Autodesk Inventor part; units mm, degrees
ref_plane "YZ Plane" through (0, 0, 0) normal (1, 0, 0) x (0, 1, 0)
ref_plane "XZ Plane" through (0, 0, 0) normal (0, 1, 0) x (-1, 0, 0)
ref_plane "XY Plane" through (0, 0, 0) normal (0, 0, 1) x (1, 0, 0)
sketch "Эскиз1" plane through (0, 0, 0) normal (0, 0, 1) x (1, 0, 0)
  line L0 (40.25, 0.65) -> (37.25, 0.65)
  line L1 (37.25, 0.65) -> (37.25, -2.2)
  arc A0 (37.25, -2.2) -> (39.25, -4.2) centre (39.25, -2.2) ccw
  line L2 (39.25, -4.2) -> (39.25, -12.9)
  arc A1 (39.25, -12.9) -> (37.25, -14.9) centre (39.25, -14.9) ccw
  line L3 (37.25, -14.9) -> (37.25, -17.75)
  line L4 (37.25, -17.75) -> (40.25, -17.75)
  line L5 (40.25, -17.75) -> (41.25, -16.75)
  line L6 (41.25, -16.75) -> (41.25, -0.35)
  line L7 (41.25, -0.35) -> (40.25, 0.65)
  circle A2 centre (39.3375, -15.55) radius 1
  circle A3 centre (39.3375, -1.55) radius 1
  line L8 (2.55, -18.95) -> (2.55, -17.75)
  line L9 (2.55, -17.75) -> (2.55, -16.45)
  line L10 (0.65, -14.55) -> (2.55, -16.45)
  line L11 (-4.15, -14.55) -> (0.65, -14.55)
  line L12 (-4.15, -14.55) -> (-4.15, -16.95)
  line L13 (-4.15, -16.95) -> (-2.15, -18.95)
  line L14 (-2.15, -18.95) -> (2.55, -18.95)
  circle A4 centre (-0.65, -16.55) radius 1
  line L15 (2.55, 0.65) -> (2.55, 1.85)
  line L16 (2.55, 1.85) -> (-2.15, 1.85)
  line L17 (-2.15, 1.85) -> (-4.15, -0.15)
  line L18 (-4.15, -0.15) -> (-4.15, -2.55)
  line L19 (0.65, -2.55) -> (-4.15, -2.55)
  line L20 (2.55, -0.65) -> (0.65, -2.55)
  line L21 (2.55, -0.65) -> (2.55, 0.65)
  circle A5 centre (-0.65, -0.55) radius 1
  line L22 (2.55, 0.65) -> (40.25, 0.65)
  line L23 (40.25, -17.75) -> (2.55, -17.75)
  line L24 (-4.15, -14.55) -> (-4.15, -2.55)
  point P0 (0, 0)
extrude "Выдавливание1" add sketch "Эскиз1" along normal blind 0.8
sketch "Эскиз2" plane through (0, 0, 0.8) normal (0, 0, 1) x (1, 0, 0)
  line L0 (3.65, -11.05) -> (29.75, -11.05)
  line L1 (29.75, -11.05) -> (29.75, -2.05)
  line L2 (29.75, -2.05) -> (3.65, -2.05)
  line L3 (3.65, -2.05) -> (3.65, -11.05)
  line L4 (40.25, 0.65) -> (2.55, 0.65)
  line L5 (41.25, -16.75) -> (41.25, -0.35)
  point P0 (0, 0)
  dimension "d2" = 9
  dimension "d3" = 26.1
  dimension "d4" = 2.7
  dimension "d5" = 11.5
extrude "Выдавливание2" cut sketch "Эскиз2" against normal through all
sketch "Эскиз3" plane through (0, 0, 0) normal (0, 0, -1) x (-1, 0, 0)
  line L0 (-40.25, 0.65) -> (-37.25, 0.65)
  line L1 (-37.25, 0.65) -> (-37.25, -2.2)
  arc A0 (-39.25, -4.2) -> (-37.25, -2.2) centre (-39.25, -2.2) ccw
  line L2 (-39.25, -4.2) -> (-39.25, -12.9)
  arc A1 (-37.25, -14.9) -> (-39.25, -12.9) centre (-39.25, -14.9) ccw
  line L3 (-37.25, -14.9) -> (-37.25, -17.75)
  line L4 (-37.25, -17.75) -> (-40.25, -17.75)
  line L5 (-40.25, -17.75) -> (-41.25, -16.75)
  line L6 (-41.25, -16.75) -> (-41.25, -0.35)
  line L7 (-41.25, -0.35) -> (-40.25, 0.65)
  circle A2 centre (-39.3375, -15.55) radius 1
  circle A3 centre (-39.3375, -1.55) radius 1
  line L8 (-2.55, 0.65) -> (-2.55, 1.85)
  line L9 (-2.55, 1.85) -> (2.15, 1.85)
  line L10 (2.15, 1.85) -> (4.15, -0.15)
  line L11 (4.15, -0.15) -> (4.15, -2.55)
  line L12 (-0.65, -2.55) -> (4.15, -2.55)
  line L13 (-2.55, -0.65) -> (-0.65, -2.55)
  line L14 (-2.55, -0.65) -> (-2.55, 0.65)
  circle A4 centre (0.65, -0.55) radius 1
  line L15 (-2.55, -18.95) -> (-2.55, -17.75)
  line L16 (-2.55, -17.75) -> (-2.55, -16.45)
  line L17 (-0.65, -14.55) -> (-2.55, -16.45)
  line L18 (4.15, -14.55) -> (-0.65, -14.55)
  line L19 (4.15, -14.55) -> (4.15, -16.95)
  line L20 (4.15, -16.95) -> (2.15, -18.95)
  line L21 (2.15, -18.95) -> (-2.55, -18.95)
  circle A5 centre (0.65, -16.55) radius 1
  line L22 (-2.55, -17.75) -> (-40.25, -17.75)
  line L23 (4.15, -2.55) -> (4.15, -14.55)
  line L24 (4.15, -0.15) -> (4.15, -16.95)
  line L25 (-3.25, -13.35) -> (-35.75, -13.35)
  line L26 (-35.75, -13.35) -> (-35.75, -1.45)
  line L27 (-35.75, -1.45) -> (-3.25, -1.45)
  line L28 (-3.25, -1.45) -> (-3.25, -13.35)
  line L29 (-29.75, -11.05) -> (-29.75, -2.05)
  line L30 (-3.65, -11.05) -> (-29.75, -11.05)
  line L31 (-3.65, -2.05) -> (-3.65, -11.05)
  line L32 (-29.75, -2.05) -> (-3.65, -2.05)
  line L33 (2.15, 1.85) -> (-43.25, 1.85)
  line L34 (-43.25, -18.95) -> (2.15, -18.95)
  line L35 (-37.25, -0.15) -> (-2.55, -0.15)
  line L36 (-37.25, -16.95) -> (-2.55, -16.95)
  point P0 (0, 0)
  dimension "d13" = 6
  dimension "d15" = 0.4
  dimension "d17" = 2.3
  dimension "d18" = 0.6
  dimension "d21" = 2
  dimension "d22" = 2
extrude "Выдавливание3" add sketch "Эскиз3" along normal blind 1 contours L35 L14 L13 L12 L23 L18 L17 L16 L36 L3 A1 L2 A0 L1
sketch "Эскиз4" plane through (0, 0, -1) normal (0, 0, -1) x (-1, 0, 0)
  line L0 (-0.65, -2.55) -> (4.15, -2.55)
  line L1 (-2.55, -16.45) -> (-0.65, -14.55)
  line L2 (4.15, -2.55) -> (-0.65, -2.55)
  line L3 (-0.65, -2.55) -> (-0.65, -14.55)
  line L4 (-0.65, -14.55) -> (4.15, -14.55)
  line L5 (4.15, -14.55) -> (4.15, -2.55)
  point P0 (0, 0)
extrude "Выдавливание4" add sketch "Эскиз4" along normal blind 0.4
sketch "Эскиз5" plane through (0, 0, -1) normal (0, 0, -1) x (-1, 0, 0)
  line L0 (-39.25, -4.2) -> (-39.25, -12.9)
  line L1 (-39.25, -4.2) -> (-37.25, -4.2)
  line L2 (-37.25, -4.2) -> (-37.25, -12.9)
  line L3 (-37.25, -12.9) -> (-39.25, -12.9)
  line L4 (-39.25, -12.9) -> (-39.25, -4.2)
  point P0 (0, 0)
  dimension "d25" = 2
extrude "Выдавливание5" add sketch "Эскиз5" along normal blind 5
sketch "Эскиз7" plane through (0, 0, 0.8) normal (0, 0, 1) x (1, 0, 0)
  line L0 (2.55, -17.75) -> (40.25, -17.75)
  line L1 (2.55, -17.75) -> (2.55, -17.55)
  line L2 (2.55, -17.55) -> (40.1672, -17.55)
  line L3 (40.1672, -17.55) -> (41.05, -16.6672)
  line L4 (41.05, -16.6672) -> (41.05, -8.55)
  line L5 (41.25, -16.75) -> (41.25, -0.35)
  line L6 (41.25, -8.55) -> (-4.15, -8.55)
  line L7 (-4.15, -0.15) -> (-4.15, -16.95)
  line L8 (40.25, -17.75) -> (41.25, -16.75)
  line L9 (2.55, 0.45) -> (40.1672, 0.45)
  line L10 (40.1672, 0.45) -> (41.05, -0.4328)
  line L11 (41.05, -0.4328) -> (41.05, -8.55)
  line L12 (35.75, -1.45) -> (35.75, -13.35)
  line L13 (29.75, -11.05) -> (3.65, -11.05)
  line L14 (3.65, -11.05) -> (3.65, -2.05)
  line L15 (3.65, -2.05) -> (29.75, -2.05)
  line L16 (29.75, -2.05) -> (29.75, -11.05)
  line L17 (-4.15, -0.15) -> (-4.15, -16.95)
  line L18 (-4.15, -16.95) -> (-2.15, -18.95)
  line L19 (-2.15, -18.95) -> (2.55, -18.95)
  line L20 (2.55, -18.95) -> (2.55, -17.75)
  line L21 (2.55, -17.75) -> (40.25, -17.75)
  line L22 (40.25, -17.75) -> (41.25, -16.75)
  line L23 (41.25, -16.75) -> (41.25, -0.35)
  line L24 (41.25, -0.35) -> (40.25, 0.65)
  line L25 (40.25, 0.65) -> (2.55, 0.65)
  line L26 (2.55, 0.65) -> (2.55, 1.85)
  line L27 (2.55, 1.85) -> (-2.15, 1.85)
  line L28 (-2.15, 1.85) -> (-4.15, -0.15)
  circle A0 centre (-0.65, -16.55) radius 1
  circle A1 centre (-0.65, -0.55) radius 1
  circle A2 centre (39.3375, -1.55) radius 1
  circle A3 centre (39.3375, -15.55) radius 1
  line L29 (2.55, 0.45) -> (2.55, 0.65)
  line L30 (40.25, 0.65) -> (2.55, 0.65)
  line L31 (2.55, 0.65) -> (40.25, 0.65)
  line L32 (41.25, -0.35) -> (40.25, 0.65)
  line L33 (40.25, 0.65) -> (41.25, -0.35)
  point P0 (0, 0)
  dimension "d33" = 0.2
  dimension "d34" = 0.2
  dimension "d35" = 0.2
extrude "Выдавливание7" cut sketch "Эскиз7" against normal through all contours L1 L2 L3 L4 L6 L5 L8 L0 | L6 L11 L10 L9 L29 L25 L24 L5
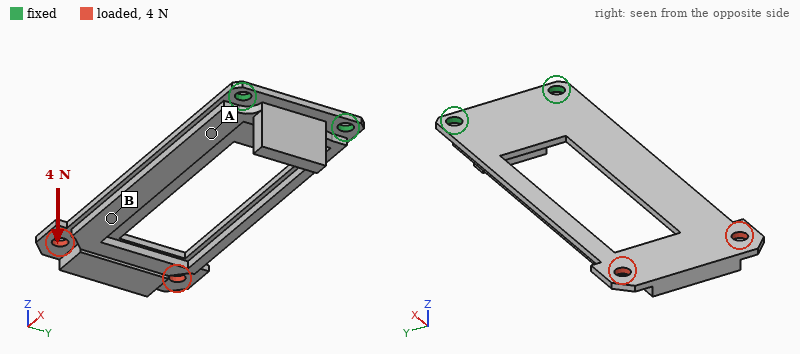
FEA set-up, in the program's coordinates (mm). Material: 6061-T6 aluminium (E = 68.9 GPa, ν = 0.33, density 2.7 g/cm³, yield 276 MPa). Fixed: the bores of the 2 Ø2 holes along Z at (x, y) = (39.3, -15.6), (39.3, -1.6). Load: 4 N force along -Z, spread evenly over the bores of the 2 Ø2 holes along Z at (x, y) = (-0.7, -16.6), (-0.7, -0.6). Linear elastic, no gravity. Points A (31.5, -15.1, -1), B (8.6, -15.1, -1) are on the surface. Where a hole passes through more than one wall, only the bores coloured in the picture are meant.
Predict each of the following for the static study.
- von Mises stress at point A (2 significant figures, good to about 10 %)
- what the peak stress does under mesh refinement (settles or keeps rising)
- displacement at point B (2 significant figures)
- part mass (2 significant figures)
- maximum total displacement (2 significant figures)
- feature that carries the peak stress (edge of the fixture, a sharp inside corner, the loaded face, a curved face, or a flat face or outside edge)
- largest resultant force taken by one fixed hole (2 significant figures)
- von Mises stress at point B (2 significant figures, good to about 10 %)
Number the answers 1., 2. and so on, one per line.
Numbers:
1. 37 MPa
2. keeps rising
3. 0.35 mm
4. 2.4 g
5. 0.60 mm
6. edge of the fixture
7. 11 N
8. 13 MPa
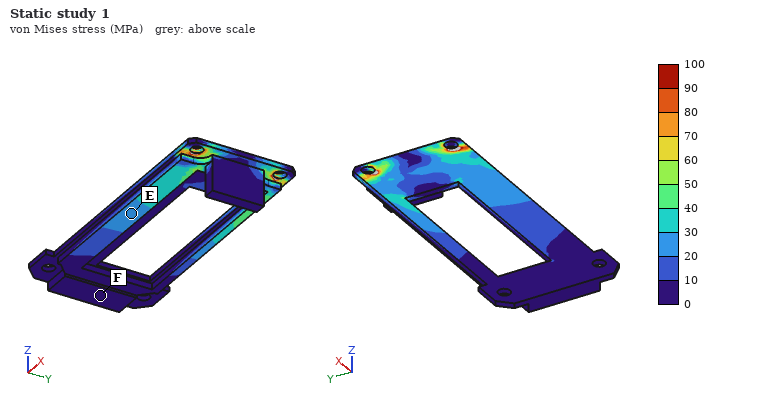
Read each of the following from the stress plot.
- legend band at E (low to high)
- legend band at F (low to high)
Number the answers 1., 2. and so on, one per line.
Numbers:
1. 20 to 30 MPa
2. 0 to 10 MPa
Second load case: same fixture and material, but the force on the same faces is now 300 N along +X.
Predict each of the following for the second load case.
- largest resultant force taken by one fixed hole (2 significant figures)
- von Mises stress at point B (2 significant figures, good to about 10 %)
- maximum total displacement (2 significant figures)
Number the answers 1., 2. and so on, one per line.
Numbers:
1. 150 N
2. 14 MPa
3. 0.38 mm
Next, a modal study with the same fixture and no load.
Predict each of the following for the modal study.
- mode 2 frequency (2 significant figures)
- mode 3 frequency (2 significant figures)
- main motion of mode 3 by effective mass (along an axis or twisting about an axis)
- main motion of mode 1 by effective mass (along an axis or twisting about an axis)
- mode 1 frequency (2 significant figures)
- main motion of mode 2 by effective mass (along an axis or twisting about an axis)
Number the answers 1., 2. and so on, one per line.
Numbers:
1. 2300 Hz
2. 3300 Hz
3. along Y
4. along Z
5. 480 Hz
6. twisting about X
